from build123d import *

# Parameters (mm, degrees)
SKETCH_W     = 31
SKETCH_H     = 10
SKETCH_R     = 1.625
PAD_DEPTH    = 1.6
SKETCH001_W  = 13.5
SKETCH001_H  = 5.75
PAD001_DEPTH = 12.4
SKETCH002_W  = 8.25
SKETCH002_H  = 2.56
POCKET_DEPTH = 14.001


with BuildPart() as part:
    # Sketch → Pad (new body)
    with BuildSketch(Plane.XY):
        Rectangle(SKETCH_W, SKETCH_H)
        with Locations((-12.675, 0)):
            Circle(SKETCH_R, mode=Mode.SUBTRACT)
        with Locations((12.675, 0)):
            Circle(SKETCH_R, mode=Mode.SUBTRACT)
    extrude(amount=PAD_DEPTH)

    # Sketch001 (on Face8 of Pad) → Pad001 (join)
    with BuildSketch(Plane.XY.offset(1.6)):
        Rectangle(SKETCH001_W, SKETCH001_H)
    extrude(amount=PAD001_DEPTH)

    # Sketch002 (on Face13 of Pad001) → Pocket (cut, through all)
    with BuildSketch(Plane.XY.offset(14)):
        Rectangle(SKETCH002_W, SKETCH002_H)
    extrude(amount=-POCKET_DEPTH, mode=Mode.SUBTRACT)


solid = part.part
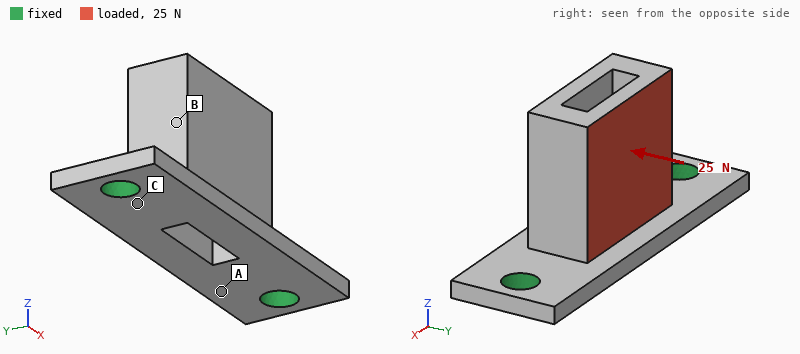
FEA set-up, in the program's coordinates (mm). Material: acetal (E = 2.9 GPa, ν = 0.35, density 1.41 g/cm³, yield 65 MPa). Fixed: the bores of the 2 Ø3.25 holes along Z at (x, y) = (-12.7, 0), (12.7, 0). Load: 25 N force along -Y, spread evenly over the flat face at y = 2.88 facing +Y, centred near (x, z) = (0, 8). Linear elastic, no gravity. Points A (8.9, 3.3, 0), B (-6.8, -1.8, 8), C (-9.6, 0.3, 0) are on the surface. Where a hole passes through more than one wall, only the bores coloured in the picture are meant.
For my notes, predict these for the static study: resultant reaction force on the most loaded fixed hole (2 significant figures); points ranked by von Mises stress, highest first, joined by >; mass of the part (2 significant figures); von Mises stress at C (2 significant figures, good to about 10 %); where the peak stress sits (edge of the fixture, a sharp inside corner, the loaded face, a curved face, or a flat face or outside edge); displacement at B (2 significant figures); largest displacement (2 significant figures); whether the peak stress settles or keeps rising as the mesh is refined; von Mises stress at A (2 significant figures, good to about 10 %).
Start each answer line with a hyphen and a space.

- 13 N
- C > A > B
- 1.6 g
- 12 MPa
- edge of the fixture
- 0.21 mm
- 0.39 mm
- keeps rising
- 6.9 MPa
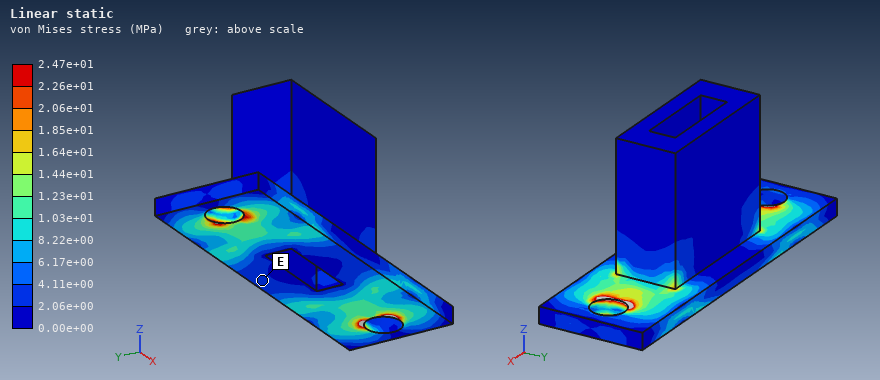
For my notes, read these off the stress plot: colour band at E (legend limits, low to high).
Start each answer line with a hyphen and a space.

- 2.06e+00 to 4.11e+00 MPa
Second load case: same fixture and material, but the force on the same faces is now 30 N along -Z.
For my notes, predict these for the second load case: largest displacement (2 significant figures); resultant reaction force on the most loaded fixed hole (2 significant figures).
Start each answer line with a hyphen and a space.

- 0.20 mm
- 17 N
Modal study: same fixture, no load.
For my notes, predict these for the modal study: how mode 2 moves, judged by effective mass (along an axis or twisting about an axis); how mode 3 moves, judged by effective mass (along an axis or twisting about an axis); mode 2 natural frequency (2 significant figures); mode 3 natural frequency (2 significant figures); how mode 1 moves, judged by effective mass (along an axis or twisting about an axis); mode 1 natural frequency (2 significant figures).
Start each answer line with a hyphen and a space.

- along Z
- along X
- 3900 Hz
- 4300 Hz
- along Y
- 1500 Hz
